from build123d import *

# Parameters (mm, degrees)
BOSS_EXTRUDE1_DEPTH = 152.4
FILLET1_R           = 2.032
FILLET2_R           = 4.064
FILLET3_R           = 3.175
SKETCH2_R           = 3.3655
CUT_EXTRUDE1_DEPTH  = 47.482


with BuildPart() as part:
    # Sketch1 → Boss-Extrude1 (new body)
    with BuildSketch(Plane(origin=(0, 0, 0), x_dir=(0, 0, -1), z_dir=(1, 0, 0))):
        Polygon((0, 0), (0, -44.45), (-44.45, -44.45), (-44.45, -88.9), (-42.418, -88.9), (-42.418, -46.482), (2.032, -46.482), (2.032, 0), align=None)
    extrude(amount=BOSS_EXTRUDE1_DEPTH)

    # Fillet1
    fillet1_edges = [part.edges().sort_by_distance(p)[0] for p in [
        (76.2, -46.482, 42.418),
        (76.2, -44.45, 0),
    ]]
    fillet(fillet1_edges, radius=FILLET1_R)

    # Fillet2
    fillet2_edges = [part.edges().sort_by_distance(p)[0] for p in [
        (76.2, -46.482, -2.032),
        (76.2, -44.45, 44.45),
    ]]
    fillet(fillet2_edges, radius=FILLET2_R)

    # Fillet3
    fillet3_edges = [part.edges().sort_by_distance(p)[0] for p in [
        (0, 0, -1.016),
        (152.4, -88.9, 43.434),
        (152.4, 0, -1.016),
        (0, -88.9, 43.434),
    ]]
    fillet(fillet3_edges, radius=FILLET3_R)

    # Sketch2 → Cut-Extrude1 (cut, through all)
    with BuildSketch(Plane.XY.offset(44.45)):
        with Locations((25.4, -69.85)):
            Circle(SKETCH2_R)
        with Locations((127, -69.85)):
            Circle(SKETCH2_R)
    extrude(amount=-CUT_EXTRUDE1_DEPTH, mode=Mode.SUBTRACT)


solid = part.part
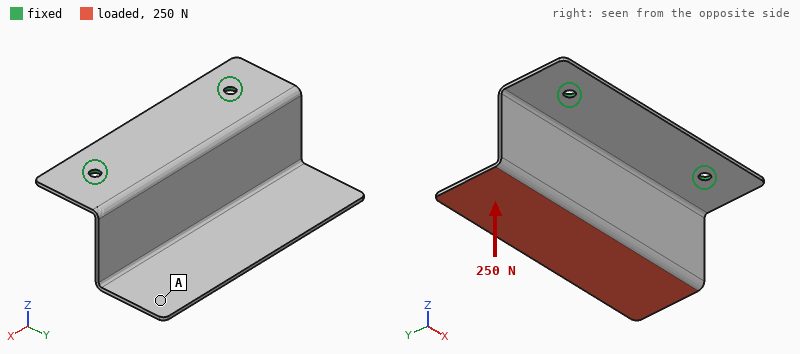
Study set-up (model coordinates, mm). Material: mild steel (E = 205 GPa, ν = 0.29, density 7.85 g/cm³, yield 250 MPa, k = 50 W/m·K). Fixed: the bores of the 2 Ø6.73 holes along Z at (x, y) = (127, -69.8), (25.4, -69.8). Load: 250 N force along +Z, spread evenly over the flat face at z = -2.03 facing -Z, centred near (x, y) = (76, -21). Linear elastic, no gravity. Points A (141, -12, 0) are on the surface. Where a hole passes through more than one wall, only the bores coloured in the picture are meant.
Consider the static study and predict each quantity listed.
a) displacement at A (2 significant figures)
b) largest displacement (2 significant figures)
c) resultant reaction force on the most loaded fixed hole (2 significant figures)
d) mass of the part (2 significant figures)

1.3 mm
1.6 mm
130 N
320 g
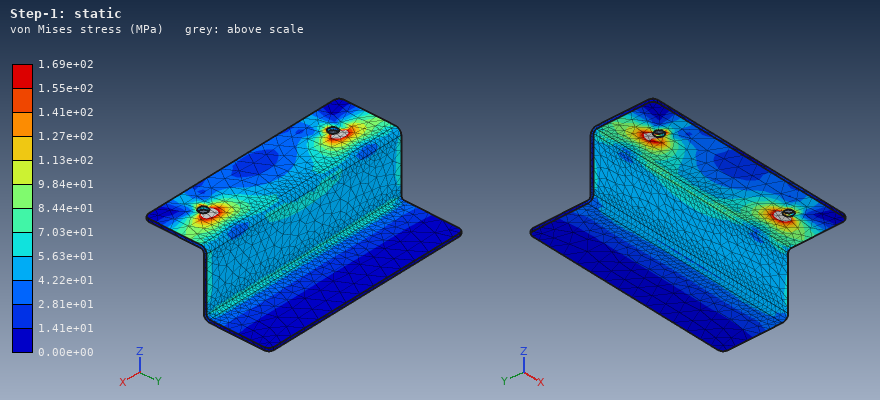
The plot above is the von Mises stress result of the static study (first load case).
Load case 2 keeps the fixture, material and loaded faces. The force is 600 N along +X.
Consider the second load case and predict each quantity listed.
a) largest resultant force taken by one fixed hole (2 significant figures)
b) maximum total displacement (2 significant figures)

480 N
0.46 mm
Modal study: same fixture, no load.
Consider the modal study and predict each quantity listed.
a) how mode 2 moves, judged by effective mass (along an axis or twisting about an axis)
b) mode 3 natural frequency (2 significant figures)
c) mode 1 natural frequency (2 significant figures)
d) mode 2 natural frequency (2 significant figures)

twisting about Z
720 Hz
170 Hz
340 Hz
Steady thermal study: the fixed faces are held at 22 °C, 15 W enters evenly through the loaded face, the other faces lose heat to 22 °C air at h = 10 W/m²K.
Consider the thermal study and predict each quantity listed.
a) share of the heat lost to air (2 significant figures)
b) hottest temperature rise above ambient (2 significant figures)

61 %
58 K
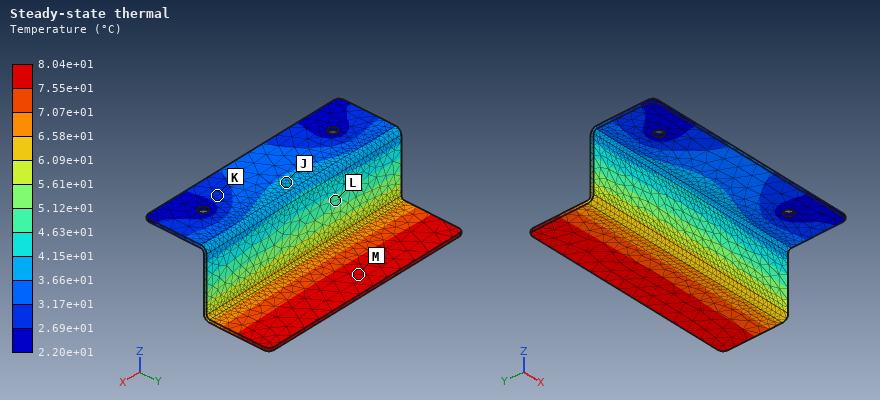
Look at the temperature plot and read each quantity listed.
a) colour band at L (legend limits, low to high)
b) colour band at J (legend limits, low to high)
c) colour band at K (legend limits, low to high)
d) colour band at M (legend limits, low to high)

4.63e+01 to 5.12e+01 °C
3.66e+01 to 4.15e+01 °C
2.69e+01 to 3.17e+01 °C
7.55e+01 to 8.04e+01 °C
